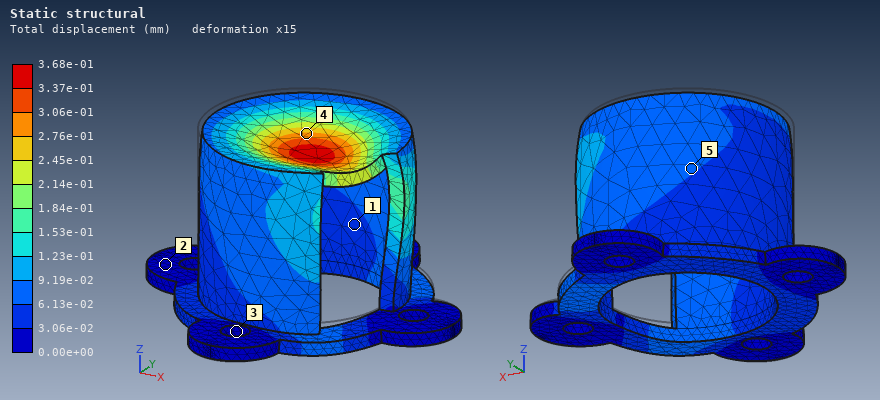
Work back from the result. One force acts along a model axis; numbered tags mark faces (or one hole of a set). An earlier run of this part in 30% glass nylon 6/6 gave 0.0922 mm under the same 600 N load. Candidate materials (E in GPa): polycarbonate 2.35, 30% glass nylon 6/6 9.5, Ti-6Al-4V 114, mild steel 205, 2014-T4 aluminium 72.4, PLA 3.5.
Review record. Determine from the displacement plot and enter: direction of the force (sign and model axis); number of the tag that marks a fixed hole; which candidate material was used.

-Z
3
polycarbonate
